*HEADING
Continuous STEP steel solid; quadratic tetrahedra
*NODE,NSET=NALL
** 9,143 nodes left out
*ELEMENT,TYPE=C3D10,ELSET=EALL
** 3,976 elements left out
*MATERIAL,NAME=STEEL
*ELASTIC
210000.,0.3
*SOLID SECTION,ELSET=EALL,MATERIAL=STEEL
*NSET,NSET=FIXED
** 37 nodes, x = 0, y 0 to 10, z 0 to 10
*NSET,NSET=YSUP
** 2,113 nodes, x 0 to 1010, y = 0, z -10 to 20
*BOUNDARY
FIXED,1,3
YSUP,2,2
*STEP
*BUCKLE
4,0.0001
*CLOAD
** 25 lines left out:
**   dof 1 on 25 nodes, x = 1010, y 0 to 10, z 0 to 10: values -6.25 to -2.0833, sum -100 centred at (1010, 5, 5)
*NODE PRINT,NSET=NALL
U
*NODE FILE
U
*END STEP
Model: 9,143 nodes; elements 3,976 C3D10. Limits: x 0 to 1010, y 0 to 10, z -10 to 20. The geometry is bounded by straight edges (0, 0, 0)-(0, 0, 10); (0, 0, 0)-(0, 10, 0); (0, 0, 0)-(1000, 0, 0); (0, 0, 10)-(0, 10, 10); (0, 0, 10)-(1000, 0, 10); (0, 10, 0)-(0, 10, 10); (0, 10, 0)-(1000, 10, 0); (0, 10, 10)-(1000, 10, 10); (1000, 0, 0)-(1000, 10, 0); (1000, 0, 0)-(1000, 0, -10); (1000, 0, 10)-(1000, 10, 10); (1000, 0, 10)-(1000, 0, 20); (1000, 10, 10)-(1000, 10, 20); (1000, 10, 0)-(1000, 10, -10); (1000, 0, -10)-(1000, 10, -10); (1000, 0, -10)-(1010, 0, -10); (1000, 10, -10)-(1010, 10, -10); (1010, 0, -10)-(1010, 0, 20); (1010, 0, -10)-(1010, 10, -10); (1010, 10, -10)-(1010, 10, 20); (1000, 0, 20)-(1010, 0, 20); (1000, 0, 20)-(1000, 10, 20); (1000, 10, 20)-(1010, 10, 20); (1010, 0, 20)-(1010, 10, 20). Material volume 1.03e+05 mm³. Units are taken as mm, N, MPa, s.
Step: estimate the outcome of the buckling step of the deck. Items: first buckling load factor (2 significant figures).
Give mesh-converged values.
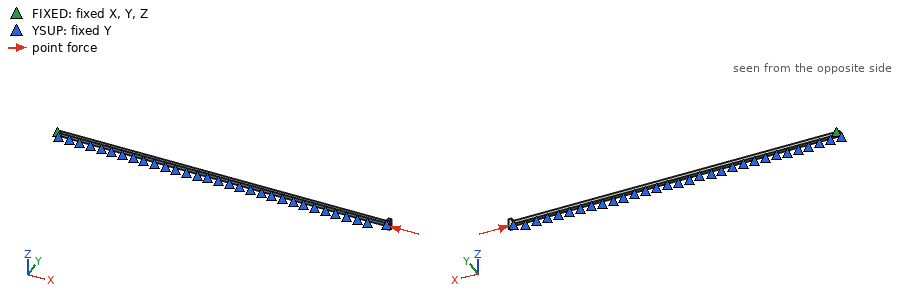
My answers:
4.2
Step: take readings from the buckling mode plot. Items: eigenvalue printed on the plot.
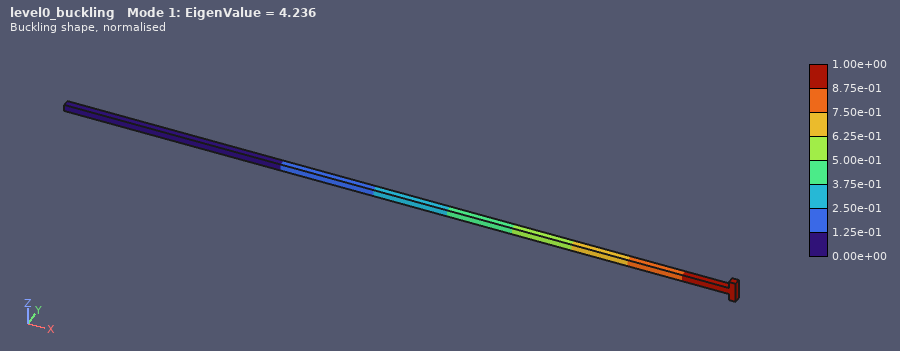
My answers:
4.236
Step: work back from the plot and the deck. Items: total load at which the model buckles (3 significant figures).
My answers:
424 N
